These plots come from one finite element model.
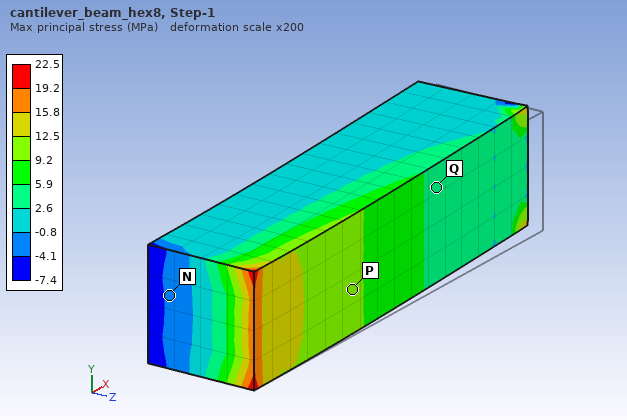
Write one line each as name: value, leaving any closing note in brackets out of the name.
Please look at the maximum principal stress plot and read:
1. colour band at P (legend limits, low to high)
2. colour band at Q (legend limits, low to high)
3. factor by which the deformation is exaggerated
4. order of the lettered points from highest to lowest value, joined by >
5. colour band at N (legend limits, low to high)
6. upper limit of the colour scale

colour band at P: 9.2 to 12.5 MPa
colour band at Q: 2.6 to 5.9 MPa
factor by which the deformation is exaggerated: 200
order of the lettered points from highest to lowest value, joined by >: P > Q > N
colour band at N: -4.1 to -0.8 MPa
upper limit of the colour scale: 22.5 MPa
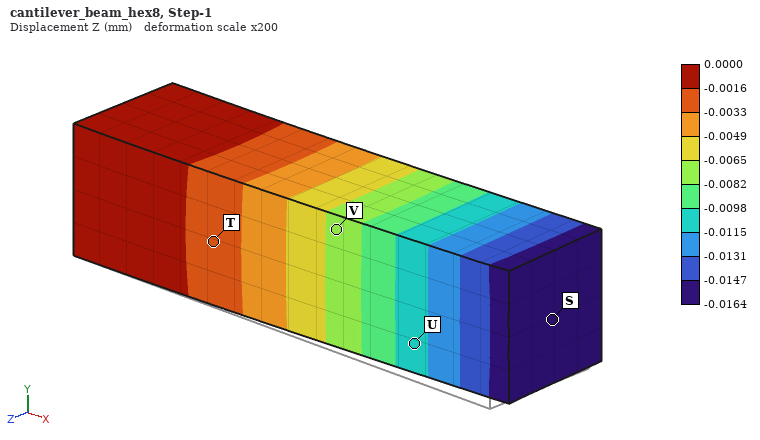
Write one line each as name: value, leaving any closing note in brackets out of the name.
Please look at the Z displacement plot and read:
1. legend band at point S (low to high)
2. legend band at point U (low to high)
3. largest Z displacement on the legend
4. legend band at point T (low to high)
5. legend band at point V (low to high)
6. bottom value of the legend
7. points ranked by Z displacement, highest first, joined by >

legend band at point S: -0.0164 to -0.0147 mm
legend band at point U: -0.0115 to -0.0098 mm
largest Z displacement on the legend: 0.0000 mm
legend band at point T: -0.0033 to -0.0016 mm
legend band at point V: -0.0082 to -0.0065 mm
bottom value of the legend: -0.0164 mm
points ranked by Z displacement, highest first, joined by >: T > V > U > S
